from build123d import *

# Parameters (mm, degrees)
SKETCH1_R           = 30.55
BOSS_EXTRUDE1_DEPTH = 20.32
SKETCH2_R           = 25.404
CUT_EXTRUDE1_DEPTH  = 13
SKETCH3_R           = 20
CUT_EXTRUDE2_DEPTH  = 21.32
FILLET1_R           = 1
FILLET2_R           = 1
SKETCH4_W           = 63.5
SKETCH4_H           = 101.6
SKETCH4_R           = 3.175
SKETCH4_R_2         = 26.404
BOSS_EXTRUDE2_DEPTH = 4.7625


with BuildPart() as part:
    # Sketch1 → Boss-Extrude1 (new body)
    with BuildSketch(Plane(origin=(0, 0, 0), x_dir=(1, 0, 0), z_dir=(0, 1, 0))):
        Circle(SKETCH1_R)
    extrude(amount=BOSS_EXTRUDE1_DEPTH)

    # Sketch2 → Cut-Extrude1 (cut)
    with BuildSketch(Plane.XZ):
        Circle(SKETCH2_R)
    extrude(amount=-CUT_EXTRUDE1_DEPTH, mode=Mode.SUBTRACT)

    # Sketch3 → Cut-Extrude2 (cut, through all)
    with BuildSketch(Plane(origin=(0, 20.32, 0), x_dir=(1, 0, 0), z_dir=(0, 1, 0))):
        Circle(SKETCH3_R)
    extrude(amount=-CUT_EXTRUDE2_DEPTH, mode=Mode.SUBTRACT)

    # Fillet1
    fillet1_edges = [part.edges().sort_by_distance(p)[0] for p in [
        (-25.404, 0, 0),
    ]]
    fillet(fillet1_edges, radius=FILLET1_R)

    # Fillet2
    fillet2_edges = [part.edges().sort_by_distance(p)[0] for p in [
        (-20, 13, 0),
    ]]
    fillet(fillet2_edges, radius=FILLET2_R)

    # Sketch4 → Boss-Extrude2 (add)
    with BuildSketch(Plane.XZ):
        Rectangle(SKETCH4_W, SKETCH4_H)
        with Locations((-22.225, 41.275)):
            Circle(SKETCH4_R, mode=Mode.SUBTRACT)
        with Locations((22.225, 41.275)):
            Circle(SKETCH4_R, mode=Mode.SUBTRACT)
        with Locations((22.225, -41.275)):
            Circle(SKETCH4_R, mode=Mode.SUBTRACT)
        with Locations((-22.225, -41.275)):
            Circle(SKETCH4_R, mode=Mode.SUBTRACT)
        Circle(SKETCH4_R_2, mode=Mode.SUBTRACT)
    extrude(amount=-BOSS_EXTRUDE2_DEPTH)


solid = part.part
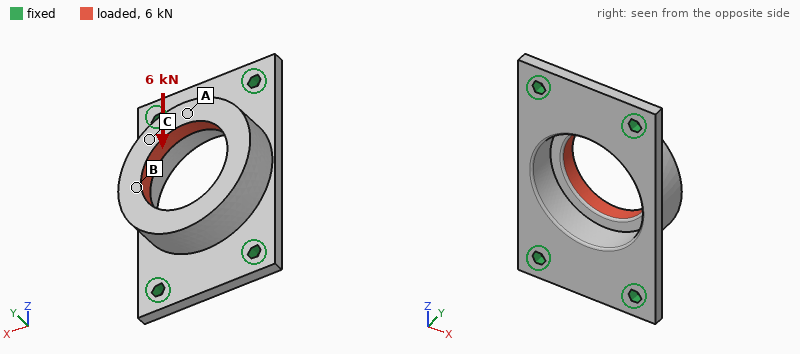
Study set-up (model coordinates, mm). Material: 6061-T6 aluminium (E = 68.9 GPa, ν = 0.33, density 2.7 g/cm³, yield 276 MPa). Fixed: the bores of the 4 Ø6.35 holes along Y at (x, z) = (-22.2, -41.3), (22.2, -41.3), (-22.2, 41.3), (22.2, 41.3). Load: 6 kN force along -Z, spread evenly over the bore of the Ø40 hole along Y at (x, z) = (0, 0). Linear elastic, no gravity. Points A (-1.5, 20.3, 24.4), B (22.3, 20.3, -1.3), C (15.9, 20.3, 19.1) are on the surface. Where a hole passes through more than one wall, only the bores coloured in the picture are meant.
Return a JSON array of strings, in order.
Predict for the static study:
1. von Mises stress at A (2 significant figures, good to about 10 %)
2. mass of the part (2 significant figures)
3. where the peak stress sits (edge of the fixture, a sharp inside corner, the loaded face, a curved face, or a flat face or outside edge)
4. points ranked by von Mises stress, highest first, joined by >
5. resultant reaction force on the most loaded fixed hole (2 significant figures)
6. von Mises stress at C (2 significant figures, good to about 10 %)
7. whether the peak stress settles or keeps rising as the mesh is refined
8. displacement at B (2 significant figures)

["22 MPa", "110 g", "edge of the fixture", "A > C > B", "1.6 kN", "16 MPa", "keeps rising", "22 µm"]
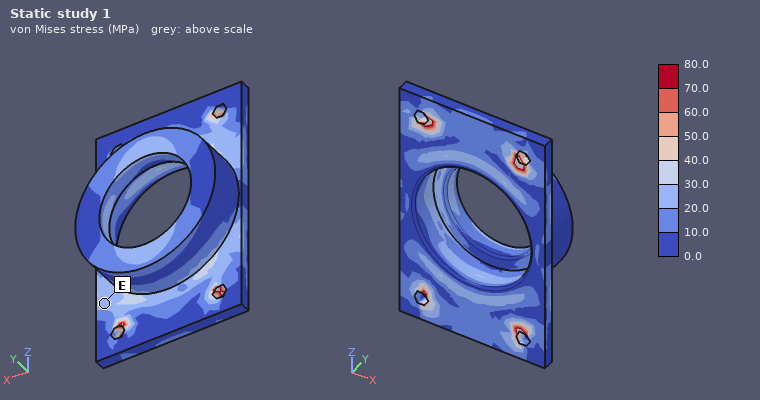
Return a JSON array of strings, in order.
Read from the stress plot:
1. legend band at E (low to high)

["20.0 to 30.0 MPa"]
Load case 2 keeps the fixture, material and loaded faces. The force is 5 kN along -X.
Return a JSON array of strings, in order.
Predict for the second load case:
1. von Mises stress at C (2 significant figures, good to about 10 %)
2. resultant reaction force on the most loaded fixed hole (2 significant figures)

["17 MPa", "1.7 kN"]
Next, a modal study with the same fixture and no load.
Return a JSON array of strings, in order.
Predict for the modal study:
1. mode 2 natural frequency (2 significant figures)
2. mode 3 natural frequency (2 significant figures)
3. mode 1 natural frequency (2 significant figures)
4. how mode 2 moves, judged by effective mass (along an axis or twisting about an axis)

["5100 Hz", "8400 Hz", "4800 Hz", "along Y"]
